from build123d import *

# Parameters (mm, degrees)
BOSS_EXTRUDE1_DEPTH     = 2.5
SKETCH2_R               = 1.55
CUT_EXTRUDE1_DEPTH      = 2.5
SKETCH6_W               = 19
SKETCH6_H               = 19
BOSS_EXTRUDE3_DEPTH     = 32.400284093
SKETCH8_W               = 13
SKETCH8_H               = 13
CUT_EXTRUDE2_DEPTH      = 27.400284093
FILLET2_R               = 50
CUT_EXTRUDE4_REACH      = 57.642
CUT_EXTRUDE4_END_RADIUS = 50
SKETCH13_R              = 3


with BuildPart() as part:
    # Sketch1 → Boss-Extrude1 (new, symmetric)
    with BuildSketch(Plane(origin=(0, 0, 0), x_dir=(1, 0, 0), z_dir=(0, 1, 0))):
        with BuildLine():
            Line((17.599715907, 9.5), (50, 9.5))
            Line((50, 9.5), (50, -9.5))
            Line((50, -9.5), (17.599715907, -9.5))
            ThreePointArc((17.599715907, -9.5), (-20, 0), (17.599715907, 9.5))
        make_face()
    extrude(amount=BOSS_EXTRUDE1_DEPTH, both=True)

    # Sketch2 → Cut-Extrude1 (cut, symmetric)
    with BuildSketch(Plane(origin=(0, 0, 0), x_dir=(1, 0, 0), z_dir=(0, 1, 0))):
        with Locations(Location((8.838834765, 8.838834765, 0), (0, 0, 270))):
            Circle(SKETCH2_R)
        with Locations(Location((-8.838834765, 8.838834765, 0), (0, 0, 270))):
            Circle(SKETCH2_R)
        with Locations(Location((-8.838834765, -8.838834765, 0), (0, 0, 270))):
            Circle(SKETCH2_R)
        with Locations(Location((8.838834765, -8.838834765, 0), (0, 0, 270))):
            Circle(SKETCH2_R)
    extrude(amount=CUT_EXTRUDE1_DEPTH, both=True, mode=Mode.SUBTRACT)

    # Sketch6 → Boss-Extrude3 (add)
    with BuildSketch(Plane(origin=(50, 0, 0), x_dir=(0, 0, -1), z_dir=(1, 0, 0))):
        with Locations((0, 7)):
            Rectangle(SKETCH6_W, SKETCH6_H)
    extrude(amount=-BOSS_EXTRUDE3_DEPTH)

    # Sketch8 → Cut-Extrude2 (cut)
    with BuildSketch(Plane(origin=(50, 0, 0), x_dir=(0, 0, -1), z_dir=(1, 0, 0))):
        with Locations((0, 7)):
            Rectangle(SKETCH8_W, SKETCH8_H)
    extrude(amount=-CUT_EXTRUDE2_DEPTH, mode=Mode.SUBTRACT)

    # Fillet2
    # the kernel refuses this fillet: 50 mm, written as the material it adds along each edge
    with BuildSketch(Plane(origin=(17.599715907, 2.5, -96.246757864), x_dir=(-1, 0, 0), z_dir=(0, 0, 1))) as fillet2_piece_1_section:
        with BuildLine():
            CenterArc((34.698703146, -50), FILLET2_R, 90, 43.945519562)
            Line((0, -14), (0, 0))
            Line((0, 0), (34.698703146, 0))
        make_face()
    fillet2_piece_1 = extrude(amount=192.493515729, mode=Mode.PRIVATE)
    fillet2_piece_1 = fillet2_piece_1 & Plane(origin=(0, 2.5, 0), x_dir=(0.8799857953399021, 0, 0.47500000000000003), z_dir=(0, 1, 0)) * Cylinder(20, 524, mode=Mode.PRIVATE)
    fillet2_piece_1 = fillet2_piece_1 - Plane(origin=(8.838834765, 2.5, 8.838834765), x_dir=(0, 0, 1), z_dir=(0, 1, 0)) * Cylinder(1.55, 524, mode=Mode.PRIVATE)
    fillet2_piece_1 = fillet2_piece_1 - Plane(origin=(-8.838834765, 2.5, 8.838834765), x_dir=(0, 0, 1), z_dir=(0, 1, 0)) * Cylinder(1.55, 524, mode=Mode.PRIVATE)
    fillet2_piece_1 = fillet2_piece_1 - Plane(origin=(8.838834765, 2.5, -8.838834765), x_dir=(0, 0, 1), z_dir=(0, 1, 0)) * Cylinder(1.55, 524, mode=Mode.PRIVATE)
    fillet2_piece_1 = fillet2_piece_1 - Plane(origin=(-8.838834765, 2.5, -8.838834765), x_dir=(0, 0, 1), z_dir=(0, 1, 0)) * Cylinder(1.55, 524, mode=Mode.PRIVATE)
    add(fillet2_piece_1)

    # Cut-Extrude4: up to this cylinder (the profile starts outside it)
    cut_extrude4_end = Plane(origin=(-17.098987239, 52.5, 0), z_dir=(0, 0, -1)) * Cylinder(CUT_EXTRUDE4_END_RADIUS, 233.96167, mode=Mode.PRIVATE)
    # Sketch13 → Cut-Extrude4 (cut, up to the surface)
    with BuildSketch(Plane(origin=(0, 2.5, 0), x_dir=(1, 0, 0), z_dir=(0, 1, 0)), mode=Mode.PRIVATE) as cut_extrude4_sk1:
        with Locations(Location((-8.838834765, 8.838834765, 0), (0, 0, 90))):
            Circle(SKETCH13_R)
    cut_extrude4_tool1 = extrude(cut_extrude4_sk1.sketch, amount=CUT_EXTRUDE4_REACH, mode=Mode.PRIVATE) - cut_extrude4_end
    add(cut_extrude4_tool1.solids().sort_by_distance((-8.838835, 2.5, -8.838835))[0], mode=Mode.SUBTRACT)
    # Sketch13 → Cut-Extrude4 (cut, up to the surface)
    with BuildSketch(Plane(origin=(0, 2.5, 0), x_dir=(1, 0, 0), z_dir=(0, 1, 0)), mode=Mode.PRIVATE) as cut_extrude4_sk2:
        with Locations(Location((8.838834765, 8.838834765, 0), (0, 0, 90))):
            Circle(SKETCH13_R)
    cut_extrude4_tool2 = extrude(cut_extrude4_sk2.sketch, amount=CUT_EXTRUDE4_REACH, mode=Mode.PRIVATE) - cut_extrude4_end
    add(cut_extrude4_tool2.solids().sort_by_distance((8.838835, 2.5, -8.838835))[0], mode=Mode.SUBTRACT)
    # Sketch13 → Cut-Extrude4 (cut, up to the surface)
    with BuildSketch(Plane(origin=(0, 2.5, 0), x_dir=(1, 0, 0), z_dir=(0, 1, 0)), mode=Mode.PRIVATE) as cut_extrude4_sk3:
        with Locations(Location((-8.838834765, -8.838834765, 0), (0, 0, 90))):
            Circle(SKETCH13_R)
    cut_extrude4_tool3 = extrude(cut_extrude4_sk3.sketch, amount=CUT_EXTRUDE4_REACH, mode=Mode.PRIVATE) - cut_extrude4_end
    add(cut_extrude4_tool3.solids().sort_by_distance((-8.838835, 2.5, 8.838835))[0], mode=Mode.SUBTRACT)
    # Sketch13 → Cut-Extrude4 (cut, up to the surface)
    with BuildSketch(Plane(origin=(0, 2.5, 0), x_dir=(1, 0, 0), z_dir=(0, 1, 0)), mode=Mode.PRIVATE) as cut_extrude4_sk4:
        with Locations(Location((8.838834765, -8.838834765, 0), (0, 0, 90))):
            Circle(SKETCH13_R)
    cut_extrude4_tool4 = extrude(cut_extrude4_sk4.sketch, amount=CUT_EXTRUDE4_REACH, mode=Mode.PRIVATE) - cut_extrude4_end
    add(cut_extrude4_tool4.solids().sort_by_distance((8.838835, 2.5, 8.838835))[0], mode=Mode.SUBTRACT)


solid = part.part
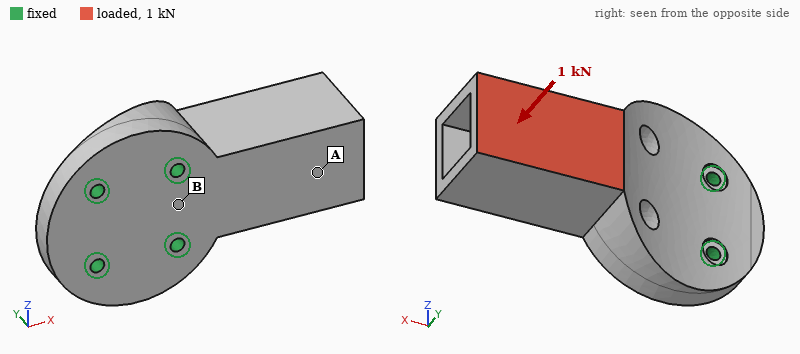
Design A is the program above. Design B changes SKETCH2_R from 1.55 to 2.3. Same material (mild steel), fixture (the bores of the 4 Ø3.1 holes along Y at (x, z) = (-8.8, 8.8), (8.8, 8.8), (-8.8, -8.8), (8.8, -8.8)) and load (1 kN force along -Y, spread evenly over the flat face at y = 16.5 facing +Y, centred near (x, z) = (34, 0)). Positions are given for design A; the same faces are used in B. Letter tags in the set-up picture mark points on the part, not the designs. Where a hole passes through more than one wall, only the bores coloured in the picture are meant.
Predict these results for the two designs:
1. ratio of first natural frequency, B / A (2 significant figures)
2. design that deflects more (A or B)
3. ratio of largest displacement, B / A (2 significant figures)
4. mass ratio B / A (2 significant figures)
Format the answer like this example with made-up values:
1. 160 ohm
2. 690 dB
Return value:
1. 1.1
2. A
3. 0.87
4. 0.99
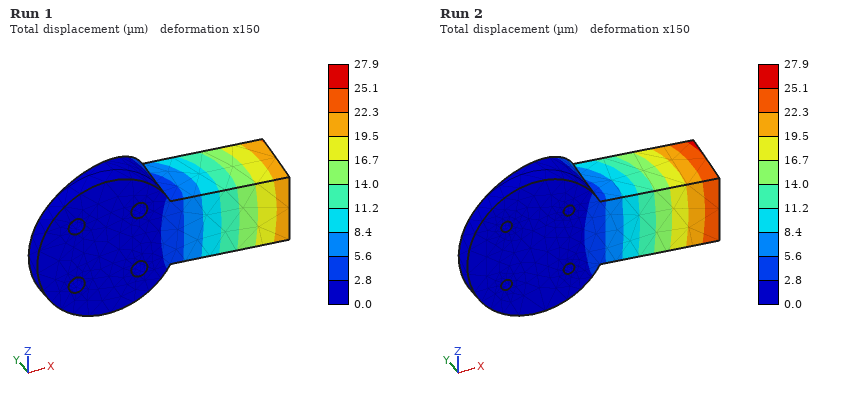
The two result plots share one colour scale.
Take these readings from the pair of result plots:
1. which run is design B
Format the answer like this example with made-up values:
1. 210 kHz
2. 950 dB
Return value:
1. Run 1
